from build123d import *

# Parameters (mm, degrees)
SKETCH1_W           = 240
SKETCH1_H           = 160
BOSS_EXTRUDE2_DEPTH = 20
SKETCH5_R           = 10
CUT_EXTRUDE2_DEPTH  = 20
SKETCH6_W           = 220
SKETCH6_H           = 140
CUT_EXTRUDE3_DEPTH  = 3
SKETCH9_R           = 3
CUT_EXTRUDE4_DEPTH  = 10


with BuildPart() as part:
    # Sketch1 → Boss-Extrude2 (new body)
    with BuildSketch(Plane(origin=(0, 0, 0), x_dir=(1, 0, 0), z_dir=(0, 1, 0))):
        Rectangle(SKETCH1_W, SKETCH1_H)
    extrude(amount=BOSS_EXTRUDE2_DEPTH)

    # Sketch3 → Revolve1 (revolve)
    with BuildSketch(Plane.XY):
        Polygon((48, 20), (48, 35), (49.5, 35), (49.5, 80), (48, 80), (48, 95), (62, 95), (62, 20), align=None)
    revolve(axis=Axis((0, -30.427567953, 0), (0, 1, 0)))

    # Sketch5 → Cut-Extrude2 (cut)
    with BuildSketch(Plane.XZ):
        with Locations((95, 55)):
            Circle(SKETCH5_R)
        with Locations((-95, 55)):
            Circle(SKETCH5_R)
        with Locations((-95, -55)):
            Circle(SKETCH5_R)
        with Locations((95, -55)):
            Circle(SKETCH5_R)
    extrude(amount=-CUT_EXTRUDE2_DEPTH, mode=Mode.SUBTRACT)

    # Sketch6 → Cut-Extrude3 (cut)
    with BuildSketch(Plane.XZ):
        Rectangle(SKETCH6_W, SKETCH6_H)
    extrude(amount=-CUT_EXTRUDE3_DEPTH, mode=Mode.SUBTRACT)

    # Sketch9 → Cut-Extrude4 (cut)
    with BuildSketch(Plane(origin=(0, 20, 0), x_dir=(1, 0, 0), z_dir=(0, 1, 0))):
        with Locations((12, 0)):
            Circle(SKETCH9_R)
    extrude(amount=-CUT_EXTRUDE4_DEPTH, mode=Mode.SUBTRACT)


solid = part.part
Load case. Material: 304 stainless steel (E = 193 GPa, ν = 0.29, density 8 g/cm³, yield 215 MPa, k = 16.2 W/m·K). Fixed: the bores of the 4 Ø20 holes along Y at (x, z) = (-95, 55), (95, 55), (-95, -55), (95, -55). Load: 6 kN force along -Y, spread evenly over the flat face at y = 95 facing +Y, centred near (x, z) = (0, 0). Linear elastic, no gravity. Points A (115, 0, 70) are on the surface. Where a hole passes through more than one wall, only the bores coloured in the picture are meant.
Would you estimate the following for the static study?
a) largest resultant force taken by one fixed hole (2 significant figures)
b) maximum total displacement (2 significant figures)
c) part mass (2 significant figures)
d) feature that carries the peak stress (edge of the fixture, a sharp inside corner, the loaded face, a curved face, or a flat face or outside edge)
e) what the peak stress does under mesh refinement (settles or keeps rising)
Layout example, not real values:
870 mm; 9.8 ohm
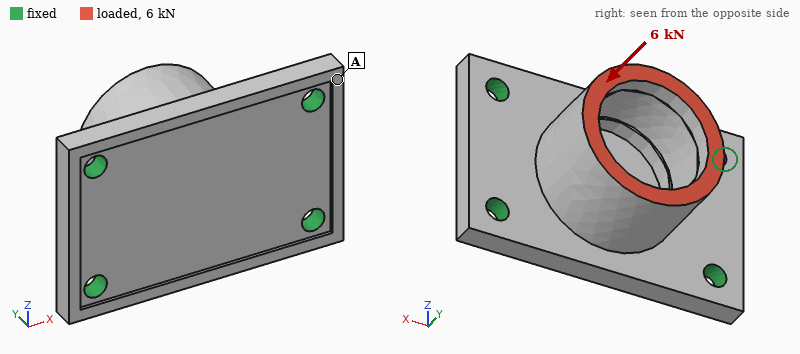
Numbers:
1.6 kN; 6.8 µm; 8.0 kg; edge of the fixture; keeps rising
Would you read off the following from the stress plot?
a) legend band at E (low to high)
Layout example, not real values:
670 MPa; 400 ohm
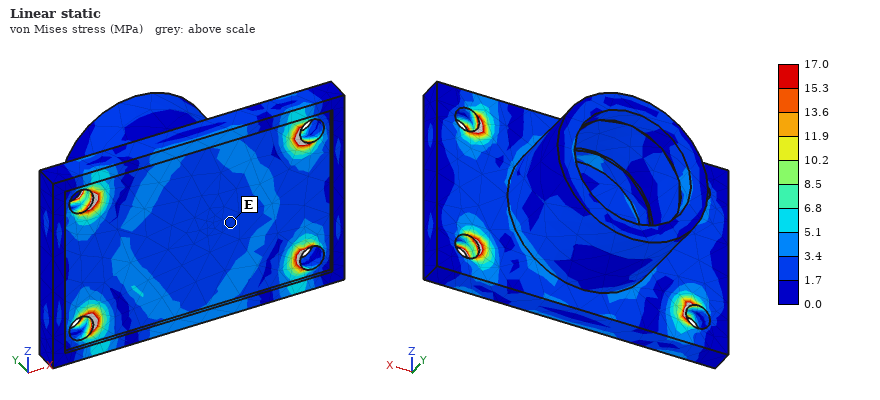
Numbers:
1.7 to 3.4 MPa
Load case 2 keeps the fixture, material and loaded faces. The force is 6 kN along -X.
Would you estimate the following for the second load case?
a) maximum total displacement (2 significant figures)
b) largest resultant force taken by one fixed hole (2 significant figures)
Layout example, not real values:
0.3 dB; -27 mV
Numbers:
12 µm; 2.3 kN
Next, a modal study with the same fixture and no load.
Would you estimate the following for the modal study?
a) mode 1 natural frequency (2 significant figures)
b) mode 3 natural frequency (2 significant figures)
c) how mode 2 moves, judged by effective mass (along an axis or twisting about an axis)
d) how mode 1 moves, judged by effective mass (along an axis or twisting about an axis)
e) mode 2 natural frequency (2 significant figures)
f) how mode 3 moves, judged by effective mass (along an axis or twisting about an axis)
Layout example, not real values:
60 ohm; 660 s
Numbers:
2000 Hz; 3100 Hz; along Y; along Z; 2200 Hz; along X
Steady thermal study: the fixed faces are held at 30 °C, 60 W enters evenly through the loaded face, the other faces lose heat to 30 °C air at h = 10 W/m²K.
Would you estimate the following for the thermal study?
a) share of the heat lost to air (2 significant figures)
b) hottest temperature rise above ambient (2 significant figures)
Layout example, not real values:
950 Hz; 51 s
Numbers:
54 %; 68 K
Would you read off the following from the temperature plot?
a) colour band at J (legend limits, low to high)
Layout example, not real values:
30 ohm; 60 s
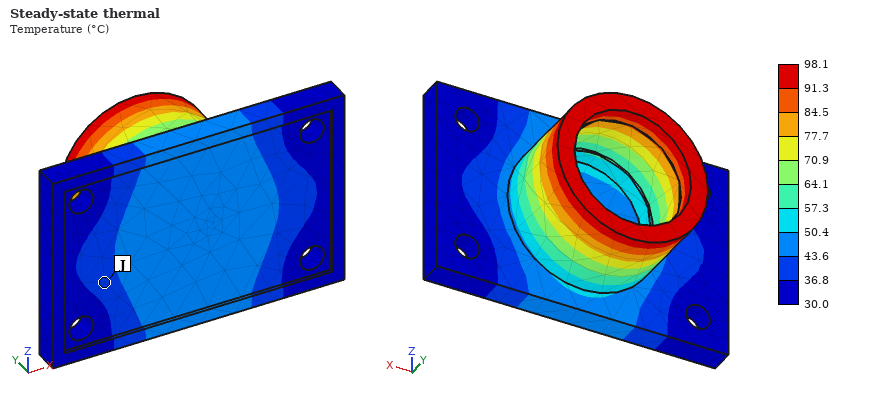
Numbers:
36.8 to 43.6 °C
